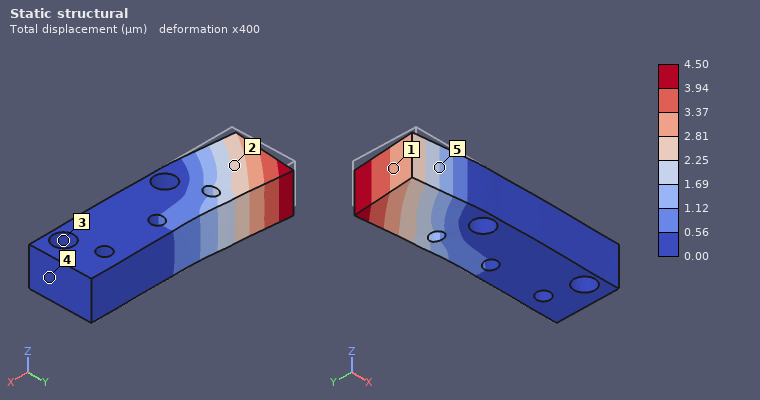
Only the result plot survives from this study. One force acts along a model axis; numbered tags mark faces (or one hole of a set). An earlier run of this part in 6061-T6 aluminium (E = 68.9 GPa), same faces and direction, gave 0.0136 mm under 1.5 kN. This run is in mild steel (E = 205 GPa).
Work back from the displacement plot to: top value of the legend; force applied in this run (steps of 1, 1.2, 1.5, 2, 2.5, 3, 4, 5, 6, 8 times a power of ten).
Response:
4.50 µm
1.5 kN
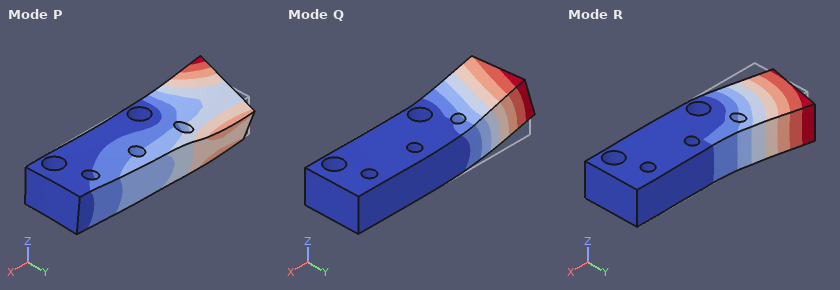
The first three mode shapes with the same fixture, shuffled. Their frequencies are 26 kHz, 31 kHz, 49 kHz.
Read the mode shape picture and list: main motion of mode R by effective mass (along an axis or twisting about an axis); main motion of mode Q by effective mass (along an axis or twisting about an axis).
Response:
along Y
along Z
